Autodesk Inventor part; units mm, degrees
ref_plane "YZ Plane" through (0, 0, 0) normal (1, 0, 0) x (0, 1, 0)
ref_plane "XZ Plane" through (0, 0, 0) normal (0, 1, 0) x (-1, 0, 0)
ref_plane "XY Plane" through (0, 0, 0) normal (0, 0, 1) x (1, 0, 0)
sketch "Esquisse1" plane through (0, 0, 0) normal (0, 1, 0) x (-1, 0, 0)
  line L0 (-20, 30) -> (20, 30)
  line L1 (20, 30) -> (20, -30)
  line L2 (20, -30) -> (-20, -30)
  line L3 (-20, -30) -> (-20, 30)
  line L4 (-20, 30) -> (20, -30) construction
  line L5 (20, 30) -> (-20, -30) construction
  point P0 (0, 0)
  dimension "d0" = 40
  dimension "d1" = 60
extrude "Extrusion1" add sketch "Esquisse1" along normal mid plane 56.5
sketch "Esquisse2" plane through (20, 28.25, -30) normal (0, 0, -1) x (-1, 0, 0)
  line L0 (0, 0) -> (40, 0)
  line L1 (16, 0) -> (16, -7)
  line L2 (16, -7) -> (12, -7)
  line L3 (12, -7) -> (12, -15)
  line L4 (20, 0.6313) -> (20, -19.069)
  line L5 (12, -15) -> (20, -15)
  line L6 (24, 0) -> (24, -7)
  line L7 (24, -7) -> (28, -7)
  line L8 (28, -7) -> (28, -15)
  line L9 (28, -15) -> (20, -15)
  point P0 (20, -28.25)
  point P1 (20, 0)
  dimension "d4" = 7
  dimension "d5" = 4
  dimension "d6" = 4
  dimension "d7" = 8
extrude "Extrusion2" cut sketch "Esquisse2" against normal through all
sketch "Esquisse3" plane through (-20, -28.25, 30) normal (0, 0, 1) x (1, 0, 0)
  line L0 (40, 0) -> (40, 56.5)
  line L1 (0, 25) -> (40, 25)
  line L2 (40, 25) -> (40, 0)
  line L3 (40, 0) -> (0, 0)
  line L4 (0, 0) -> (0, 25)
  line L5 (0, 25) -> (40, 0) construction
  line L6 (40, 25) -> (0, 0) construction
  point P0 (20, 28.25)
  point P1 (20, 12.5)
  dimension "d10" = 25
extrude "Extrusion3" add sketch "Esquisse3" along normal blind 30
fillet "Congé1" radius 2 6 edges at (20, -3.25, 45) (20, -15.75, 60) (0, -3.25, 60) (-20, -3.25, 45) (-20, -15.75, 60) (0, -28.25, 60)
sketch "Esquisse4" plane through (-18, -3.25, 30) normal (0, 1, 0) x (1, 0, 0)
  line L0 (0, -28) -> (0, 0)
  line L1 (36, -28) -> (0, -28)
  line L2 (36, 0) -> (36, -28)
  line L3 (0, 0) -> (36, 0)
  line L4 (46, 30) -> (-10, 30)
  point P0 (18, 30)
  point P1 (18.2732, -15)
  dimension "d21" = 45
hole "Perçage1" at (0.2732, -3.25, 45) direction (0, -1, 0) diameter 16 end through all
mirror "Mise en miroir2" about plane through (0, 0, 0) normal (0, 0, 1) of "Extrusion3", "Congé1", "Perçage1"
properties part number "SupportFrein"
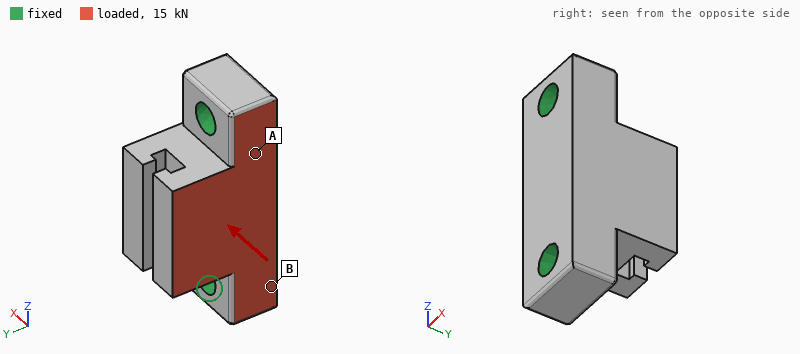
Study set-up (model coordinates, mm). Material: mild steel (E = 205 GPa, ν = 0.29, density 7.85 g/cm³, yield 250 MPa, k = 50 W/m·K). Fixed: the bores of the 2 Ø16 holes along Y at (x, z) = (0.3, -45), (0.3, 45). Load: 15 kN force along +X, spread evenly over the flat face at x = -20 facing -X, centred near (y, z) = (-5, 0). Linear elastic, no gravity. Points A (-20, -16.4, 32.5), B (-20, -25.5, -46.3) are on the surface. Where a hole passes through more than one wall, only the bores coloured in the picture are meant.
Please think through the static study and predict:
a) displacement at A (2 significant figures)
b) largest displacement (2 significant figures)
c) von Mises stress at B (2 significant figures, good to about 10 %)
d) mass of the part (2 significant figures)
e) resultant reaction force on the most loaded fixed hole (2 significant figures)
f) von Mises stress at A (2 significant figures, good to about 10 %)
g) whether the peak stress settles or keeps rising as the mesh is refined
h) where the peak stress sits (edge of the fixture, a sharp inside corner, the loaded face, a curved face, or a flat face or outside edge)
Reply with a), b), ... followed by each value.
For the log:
a) 2.2 µm
b) 14 µm
c) 6.8 MPa
d) 1.4 kg
e) 7.5 kN
f) 19 MPa
g) keeps rising
h) edge of the fixture
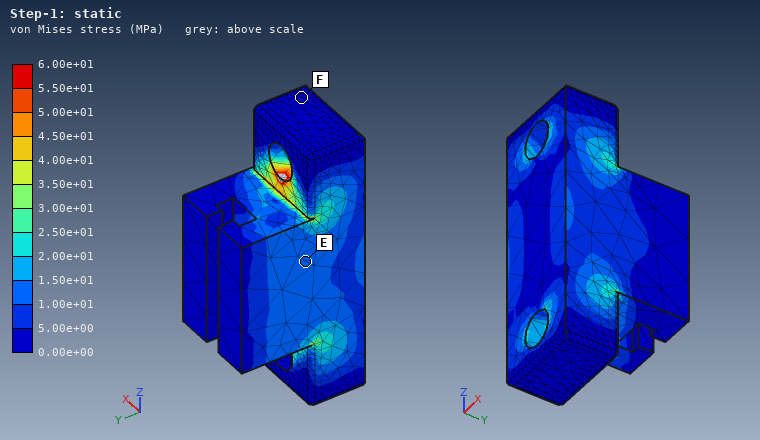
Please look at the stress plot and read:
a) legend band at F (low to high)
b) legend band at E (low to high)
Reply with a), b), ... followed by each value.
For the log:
a) 0.00e+00 to 5.00e+00 MPa
b) 1.00e+01 to 1.50e+01 MPa
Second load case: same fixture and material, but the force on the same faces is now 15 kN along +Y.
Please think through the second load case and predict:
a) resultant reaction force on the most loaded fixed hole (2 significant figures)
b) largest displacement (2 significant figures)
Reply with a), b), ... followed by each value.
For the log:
a) 7.7 kN
b) 15 µm
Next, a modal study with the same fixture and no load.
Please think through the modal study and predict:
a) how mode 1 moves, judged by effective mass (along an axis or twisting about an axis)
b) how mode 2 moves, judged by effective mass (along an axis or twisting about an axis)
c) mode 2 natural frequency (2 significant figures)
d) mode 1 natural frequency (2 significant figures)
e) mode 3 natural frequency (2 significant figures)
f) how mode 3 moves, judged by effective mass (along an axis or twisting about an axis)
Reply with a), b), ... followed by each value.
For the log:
a) along X
b) along Y
c) 11 kHz
d) 6100 Hz
e) 13 kHz
f) along Z
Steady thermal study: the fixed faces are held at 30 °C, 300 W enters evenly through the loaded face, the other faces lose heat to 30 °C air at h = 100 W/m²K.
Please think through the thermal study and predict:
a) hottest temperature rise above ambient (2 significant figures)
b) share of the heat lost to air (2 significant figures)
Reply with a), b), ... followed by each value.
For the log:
a) 80 K
b) 20 %
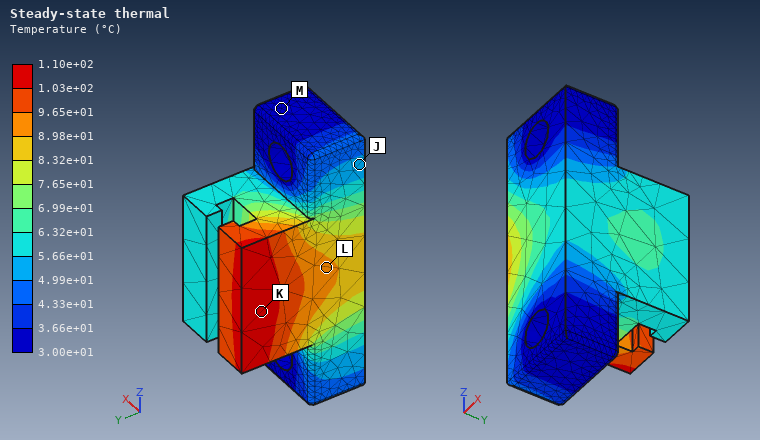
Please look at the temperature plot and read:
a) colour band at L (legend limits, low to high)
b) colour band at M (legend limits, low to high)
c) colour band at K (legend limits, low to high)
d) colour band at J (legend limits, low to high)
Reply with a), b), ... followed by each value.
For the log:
a) 8.98e+01 to 9.65e+01 °C
b) 3.00e+01 to 3.66e+01 °C
c) 1.03e+02 to 1.10e+02 °C
d) 4.99e+01 to 5.66e+01 °C
